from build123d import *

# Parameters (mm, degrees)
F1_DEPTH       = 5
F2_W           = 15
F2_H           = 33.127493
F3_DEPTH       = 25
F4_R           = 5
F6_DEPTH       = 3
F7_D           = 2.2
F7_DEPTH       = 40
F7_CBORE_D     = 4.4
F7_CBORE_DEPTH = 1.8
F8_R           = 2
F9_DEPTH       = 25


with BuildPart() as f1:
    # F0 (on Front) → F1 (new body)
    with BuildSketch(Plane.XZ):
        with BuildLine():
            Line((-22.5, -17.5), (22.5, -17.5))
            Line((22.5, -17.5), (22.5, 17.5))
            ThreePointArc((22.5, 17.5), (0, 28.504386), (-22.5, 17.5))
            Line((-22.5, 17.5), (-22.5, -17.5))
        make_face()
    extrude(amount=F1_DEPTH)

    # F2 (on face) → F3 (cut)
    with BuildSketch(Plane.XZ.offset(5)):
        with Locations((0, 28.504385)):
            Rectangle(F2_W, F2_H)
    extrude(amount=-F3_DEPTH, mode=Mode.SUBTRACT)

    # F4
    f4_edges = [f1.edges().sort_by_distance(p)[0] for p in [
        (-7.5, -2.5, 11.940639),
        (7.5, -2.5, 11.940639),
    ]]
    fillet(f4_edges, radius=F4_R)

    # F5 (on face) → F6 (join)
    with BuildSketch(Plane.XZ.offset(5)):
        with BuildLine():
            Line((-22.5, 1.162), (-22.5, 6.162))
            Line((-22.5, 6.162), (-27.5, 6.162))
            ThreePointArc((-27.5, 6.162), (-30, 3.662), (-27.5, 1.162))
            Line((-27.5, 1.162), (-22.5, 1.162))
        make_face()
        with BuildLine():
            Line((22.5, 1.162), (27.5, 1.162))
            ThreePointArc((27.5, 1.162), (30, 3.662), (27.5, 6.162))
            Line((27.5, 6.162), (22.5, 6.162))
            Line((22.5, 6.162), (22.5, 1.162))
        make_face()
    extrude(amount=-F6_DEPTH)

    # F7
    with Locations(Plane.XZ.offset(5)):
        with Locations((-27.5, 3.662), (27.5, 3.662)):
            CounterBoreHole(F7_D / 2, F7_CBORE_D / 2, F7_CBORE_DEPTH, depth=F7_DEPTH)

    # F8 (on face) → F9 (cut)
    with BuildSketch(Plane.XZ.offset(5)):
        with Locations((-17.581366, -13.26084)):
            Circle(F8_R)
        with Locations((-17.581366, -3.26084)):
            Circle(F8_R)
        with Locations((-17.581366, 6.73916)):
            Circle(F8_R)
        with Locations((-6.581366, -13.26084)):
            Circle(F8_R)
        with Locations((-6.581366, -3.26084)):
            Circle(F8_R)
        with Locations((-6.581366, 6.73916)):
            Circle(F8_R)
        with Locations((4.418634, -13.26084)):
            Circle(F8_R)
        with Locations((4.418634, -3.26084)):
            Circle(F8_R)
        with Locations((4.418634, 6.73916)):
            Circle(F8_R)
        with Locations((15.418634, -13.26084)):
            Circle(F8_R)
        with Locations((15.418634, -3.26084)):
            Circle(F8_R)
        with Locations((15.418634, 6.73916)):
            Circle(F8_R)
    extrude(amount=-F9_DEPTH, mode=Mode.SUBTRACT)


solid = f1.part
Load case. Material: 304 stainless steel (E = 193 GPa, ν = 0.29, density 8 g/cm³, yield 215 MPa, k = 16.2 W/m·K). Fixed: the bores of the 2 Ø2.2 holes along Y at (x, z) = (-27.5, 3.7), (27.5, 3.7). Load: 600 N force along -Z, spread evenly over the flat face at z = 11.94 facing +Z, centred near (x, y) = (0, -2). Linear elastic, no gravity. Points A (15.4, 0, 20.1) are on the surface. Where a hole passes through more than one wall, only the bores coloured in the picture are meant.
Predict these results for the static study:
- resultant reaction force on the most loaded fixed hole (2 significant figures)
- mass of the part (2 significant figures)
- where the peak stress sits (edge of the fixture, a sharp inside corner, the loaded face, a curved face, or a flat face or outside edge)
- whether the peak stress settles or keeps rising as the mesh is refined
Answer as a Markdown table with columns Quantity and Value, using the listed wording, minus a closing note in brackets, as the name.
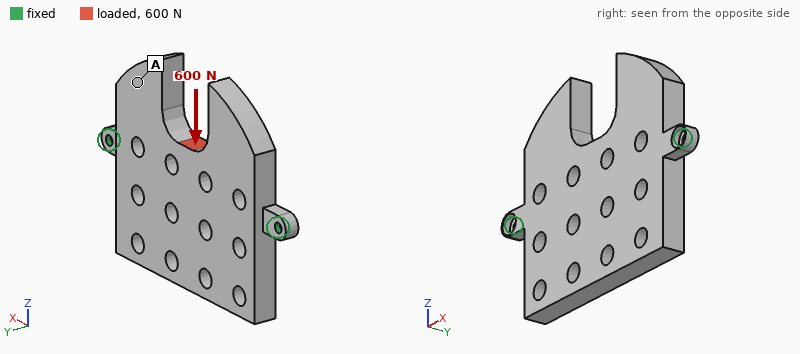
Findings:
| Quantity | Value |
|---|---|
| resultant reaction force on the most loaded fixed hole | 300 N |
| mass of the part | 63 g |
| where the peak stress sits | edge of the fixture |
| whether the peak stress settles or keeps rising as the mesh is refined | keeps rising |
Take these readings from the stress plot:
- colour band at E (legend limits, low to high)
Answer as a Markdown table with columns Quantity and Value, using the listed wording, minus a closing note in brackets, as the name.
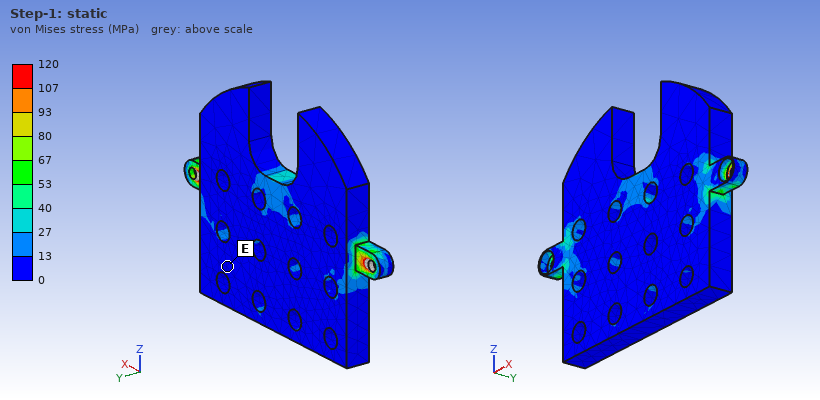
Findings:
| Quantity | Value |
|---|---|
| colour band at E | 0 to 13 MPa |
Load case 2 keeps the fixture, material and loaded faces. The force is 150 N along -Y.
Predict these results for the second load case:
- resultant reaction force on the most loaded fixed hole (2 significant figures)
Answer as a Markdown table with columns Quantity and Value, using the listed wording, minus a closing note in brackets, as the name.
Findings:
| Quantity | Value |
|---|---|
| resultant reaction force on the most loaded fixed hole | 75 N |
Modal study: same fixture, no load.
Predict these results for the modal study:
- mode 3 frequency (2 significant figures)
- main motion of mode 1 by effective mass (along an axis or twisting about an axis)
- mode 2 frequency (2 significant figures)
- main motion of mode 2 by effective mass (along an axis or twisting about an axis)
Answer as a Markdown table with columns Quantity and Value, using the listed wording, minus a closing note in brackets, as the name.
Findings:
| Quantity | Value |
|---|---|
| mode 3 frequency | 5900 Hz |
| main motion of mode 1 by effective mass | twisting about X |
| mode 2 frequency | 2900 Hz |
| main motion of mode 2 by effective mass | along Y |
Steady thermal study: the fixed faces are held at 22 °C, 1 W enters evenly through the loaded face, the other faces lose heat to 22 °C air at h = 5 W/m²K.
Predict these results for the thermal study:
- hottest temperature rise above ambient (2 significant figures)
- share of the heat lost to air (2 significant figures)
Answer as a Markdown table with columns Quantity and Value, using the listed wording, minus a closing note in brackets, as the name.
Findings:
| Quantity | Value |
|---|---|
| hottest temperature rise above ambient | 25 K |
| share of the heat lost to air | 33 % |
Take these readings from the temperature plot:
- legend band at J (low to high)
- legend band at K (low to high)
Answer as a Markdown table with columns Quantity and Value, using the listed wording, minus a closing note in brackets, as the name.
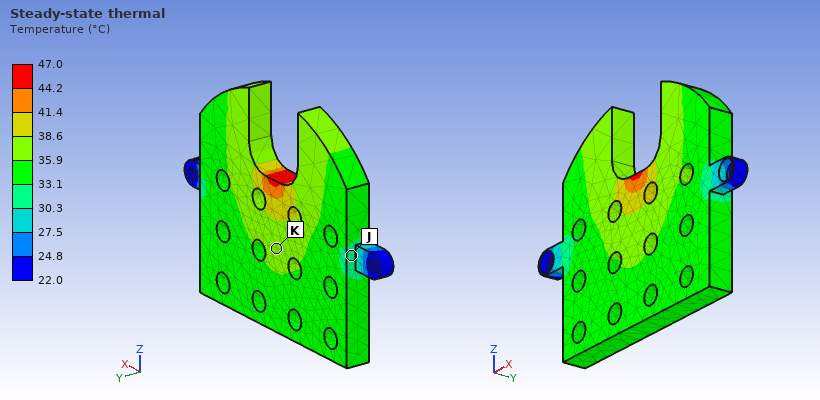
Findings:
| Quantity | Value |
|---|---|
| legend band at J | 30.3 to 33.1 °C |
| legend band at K | 35.9 to 38.6 °C |
